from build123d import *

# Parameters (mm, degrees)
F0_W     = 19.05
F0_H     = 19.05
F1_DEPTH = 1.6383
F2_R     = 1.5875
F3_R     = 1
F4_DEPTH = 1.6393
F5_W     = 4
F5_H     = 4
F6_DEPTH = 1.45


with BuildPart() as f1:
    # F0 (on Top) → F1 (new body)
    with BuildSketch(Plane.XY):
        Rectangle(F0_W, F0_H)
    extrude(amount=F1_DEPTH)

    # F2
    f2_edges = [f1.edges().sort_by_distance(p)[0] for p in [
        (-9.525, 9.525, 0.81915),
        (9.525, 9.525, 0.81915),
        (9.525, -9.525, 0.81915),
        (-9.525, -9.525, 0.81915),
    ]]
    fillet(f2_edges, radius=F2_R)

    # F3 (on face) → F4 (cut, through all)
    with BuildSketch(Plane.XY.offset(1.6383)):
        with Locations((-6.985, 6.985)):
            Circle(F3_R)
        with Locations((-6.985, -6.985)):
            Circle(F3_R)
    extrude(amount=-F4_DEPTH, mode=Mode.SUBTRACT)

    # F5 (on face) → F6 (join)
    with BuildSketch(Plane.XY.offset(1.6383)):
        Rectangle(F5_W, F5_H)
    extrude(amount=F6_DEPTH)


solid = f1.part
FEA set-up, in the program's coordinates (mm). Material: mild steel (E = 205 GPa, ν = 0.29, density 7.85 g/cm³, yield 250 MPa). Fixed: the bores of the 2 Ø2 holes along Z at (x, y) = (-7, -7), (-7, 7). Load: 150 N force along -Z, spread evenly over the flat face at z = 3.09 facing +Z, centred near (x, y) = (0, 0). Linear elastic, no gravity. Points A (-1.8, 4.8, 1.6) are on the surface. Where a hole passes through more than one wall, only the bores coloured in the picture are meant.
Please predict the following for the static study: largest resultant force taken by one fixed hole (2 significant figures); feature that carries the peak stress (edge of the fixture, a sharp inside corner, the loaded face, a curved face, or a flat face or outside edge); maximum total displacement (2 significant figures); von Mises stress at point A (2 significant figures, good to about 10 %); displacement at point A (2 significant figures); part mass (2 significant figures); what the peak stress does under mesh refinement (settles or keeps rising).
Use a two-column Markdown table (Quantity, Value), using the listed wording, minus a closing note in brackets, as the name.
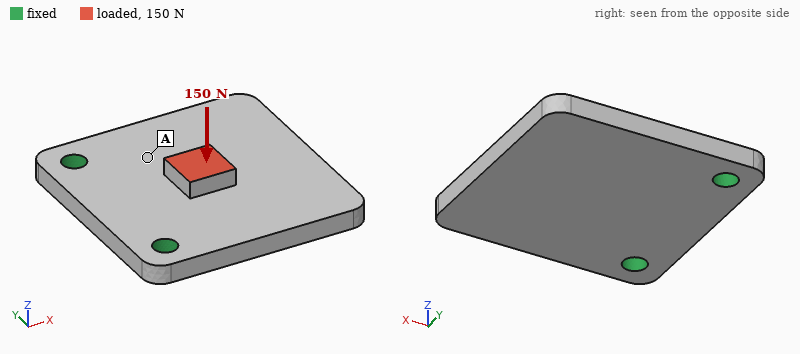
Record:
| Quantity | Value |
|---|---|
| largest resultant force taken by one fixed hole | 75 N |
| feature that carries the peak stress | edge of the fixture |
| maximum total displacement | 46 µm |
| von Mises stress at point A | 33 MPa |
| displacement at point A | 10 µm |
| part mass | 4.7 g |
| what the peak stress does under mesh refinement | keeps rising |
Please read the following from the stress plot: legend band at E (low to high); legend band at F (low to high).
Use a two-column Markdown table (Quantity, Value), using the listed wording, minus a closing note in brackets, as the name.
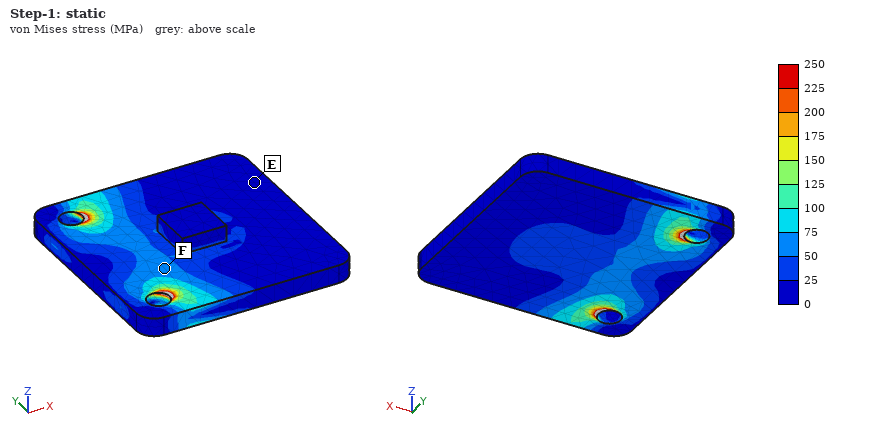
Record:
| Quantity | Value |
|---|---|
| legend band at E | 0 to 25 MPa |
| legend band at F | 50 to 75 MPa |
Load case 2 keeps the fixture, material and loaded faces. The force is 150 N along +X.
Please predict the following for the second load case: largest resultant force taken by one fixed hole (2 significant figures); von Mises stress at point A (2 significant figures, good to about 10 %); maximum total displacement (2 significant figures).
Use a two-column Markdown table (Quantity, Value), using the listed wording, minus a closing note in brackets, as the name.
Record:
| Quantity | Value |
|---|---|
| largest resultant force taken by one fixed hole | 79 N |
| von Mises stress at point A | 34 MPa |
| maximum total displacement | 22 µm |
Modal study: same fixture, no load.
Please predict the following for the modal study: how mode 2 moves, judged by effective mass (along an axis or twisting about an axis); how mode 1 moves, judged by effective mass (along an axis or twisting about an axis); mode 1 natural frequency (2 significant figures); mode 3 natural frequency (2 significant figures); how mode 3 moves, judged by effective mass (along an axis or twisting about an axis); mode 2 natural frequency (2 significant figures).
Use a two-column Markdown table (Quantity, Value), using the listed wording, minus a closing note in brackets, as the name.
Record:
| Quantity | Value |
|---|---|
| how mode 2 moves, judged by effective mass | twisting about X |
| how mode 1 moves, judged by effective mass | along Z |
| mode 1 natural frequency | 4800 Hz |
| mode 3 natural frequency | 28 kHz |
| how mode 3 moves, judged by effective mass | along Z |
| mode 2 natural frequency | 12 kHz |
